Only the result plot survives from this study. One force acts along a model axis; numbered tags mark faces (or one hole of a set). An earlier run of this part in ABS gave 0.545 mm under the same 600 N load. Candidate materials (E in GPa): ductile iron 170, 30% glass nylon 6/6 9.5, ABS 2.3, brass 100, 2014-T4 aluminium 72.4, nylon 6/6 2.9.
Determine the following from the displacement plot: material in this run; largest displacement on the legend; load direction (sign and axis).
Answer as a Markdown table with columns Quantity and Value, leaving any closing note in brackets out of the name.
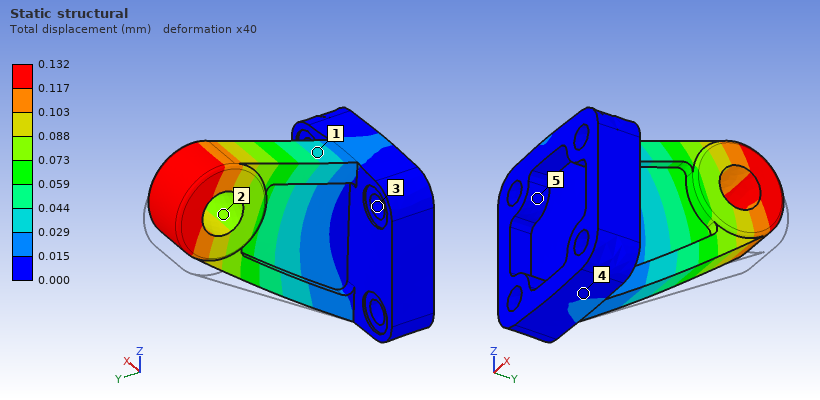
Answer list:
| Quantity | Value |
|---|---|
| material in this run | 30% glass nylon 6/6 |
| largest displacement on the legend | 0.132 mm |
| load direction | +Z |
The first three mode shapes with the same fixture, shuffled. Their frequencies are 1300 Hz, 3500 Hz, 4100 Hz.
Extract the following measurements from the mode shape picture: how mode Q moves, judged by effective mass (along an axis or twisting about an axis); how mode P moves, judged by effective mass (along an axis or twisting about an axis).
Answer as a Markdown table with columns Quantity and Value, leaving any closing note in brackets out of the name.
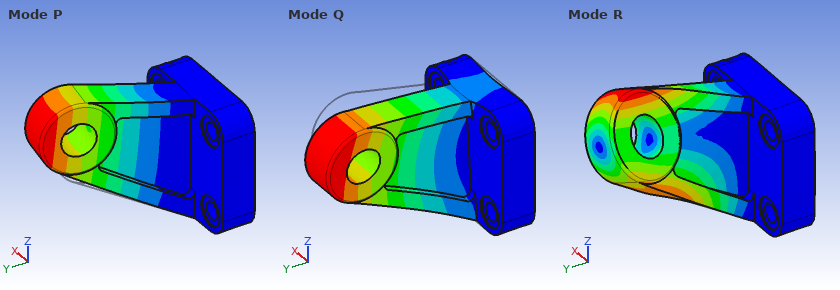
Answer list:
| Quantity | Value |
|---|---|
| how mode Q moves, judged by effective mass | along Z |
| how mode P moves, judged by effective mass | along X |
